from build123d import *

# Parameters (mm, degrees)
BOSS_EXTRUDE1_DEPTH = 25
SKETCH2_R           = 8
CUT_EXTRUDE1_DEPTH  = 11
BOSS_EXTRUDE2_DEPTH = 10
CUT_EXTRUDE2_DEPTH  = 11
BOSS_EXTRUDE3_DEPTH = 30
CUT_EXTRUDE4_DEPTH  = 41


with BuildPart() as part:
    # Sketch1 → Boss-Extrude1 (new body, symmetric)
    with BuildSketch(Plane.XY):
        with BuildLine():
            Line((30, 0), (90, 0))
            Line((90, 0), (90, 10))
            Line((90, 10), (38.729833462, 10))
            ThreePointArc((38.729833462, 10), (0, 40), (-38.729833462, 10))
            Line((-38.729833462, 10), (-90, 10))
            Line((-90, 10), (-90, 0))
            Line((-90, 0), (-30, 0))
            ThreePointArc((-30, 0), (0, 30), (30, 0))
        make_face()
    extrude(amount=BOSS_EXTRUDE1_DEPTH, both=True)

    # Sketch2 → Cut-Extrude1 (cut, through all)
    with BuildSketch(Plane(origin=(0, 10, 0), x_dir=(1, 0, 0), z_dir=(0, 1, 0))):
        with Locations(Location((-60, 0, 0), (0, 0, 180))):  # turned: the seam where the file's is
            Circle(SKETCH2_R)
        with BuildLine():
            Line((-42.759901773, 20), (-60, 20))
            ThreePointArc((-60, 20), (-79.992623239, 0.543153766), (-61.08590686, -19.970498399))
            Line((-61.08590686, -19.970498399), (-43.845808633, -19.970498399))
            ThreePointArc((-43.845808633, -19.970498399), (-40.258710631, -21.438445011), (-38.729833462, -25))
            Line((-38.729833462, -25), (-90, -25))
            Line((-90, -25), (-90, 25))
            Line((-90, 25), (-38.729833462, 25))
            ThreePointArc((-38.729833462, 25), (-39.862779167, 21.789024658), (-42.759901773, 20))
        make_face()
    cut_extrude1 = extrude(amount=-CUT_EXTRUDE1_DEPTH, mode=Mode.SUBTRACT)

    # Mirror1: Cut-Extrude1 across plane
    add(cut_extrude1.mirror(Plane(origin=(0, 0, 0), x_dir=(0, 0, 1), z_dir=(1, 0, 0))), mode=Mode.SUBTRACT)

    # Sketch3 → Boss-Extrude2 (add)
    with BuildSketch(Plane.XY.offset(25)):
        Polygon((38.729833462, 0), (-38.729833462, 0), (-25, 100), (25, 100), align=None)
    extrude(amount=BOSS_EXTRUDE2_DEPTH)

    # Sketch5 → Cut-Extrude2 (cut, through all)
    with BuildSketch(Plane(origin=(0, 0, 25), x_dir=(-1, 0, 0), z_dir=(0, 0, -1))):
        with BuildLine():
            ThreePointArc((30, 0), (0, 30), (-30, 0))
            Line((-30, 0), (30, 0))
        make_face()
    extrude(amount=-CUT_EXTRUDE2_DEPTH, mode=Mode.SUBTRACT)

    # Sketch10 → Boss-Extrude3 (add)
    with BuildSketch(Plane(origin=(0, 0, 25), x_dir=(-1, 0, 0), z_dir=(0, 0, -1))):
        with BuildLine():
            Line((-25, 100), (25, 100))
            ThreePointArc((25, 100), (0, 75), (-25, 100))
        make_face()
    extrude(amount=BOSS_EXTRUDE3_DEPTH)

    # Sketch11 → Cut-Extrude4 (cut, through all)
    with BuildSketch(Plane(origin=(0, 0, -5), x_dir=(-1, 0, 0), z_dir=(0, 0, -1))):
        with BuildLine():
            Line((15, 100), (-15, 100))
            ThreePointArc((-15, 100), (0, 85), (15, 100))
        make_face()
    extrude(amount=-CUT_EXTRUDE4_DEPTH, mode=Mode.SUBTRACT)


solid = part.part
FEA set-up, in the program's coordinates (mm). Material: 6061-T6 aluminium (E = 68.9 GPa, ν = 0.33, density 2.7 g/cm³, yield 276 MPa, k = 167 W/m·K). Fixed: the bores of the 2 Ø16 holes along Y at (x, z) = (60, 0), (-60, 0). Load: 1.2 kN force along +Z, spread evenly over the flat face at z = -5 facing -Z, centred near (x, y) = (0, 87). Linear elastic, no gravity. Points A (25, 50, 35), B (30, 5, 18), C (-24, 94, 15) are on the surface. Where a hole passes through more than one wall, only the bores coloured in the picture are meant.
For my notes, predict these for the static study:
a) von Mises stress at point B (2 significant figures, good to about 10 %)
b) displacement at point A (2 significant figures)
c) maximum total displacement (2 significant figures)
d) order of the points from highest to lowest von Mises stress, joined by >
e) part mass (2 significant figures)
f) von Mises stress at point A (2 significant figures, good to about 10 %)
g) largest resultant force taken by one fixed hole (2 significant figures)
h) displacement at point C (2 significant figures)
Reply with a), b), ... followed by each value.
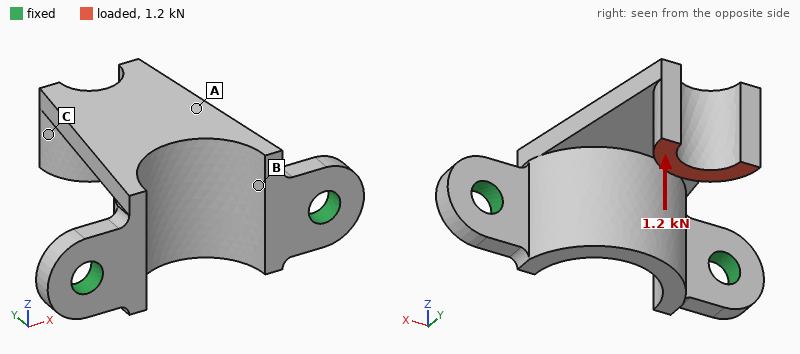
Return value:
a) 16 MPa
b) 0.18 mm
c) 0.55 mm
d) A > B > C
e) 390 g
f) 42 MPa
g) 680 N
h) 0.46 mm
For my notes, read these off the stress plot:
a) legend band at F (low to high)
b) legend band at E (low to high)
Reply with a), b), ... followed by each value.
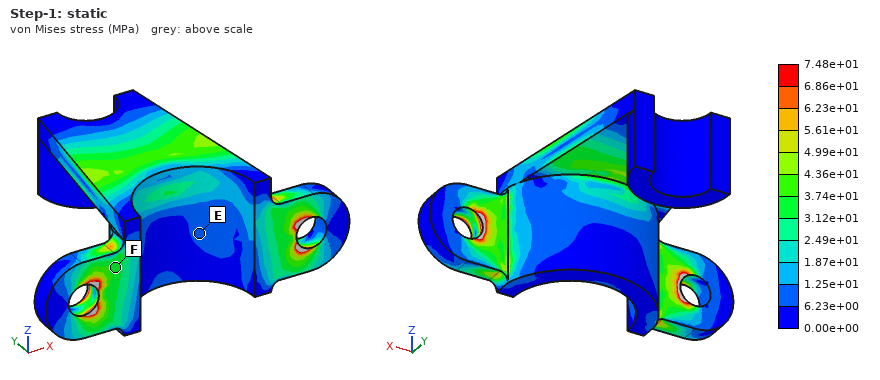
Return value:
a) 3.12e+01 to 3.74e+01 MPa
b) 6.23e+00 to 1.25e+01 MPa
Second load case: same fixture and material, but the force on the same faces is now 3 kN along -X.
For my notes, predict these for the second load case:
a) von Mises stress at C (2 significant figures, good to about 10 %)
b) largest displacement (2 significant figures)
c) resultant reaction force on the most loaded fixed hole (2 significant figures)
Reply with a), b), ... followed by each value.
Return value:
a) 21 MPa
b) 0.60 mm
c) 3.2 kN
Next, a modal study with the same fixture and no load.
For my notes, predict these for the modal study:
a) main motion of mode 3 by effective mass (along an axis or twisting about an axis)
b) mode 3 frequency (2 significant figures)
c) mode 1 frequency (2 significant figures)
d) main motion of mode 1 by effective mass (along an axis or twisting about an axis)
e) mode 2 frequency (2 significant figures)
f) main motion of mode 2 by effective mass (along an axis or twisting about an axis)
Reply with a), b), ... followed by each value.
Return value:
a) along Y
b) 2100 Hz
c) 840 Hz
d) along Z
e) 1900 Hz
f) along X
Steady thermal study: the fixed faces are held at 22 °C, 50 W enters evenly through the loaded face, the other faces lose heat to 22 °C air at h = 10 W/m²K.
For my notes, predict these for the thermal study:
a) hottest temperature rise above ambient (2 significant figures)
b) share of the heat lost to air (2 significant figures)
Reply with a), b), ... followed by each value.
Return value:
a) 56 K
b) 13 %
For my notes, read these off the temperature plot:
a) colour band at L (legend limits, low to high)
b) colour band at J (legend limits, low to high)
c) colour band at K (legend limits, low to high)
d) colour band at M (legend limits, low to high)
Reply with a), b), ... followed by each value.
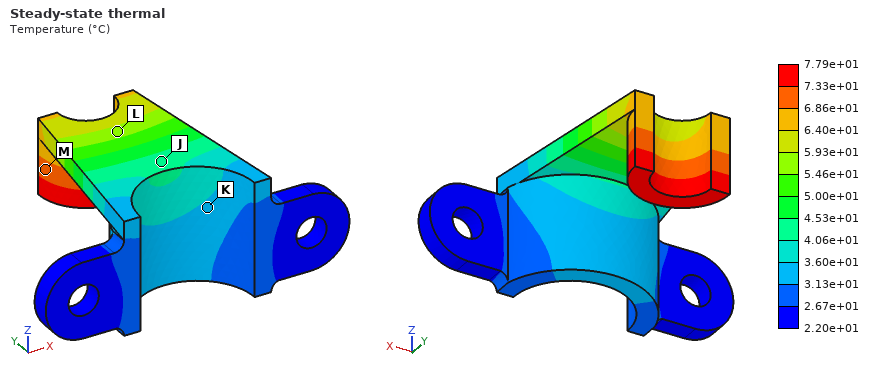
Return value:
a) 5.46e+01 to 5.93e+01 °C
b) 4.06e+01 to 4.53e+01 °C
c) 3.13e+01 to 3.60e+01 °C
d) 6.86e+01 to 7.33e+01 °C
